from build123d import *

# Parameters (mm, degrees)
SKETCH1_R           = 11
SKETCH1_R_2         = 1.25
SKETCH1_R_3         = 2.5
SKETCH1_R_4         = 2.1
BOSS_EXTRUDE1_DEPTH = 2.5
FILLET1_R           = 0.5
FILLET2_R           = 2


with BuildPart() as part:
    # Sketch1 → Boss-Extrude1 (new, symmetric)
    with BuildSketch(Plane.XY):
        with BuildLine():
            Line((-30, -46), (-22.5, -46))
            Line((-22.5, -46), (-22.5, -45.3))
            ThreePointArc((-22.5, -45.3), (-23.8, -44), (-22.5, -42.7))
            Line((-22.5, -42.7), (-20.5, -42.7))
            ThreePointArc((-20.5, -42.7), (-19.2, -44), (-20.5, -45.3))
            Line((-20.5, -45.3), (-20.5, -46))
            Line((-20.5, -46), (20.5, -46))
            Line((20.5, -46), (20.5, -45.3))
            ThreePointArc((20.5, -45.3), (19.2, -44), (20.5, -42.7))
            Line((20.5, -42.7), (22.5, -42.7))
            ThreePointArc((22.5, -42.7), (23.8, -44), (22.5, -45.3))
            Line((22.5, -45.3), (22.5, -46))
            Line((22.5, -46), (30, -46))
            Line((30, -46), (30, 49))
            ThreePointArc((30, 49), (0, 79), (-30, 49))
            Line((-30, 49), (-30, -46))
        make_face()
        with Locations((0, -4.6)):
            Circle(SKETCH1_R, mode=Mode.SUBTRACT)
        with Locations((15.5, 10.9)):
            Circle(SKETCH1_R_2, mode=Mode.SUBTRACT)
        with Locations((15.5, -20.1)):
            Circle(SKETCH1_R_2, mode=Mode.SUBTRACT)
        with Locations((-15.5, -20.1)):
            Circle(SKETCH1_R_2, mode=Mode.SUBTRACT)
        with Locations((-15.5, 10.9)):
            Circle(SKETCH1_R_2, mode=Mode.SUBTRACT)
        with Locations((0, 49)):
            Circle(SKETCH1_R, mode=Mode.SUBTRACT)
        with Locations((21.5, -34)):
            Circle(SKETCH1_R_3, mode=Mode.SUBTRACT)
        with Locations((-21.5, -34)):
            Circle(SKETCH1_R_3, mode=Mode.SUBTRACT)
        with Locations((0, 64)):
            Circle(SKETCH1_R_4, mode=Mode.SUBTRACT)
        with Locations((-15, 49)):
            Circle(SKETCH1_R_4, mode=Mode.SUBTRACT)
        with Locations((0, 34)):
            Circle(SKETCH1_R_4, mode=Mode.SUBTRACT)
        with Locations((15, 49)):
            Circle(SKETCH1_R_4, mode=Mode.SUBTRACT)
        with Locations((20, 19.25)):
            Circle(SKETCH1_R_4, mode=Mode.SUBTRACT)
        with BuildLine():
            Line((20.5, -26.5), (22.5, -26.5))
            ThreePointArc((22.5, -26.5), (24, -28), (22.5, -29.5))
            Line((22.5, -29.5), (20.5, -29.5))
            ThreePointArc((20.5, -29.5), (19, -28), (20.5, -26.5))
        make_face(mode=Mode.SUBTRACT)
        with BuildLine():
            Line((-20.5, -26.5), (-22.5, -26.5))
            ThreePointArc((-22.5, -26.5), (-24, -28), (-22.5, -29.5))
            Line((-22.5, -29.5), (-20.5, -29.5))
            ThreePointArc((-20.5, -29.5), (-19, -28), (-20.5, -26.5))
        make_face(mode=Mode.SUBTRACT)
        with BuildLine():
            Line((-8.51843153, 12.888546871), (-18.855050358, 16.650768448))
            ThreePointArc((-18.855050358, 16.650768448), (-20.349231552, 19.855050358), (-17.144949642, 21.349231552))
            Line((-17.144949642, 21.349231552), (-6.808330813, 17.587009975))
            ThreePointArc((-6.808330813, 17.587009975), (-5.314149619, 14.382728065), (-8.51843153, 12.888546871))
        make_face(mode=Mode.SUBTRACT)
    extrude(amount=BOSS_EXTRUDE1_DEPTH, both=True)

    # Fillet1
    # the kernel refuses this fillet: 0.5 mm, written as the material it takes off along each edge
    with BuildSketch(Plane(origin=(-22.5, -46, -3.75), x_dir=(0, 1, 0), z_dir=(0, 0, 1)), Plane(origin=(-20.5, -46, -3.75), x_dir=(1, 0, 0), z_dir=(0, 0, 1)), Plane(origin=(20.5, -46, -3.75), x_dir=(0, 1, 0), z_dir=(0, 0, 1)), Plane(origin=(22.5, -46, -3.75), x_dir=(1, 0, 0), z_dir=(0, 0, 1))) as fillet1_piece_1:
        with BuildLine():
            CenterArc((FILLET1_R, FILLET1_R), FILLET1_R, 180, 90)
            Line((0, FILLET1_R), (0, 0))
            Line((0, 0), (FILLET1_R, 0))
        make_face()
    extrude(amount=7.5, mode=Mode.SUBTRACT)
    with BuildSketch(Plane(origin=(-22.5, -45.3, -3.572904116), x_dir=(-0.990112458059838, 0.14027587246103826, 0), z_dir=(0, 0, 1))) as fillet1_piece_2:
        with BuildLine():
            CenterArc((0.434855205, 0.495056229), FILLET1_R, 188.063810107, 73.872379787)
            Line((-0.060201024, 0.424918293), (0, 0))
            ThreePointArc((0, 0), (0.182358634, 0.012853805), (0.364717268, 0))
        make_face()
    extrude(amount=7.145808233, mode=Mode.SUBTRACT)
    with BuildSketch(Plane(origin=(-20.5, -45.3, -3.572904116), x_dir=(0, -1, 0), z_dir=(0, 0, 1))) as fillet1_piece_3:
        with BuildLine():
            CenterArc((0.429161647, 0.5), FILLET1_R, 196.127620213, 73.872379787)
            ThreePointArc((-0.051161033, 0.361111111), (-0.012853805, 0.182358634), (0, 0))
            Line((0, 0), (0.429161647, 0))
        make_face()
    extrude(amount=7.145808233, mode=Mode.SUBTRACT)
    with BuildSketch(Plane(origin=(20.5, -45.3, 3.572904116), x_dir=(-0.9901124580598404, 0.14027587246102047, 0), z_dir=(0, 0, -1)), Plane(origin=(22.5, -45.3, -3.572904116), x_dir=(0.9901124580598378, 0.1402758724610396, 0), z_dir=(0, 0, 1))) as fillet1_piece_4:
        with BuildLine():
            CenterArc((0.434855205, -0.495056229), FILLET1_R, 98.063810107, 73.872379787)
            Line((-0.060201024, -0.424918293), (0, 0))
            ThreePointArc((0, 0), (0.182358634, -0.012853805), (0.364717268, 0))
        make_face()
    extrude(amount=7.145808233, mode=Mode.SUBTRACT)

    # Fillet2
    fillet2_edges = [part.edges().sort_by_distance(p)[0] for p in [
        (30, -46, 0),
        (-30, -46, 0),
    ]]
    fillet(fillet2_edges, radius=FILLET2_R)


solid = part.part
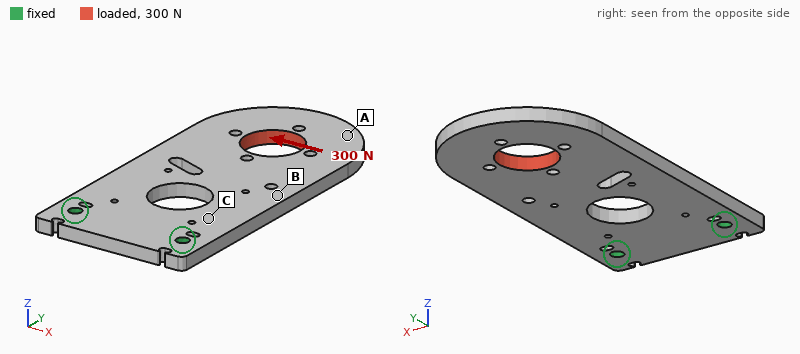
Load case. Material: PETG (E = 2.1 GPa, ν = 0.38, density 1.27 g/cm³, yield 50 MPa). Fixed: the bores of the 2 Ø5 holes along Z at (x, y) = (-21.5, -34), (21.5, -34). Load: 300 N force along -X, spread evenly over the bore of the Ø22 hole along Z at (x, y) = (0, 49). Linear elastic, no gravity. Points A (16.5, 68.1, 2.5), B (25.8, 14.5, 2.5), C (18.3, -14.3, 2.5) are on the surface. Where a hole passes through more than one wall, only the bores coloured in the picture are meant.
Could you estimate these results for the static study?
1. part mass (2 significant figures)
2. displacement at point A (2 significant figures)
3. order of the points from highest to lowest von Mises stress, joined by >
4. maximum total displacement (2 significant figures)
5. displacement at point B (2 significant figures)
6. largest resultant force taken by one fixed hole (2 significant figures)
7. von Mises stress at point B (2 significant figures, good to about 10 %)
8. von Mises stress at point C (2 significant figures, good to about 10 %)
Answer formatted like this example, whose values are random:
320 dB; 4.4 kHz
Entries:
39 g; 0.83 mm; C > B > A; 0.90 mm; 0.38 mm; 570 N; 2.8 MPa; 4.9 MPa
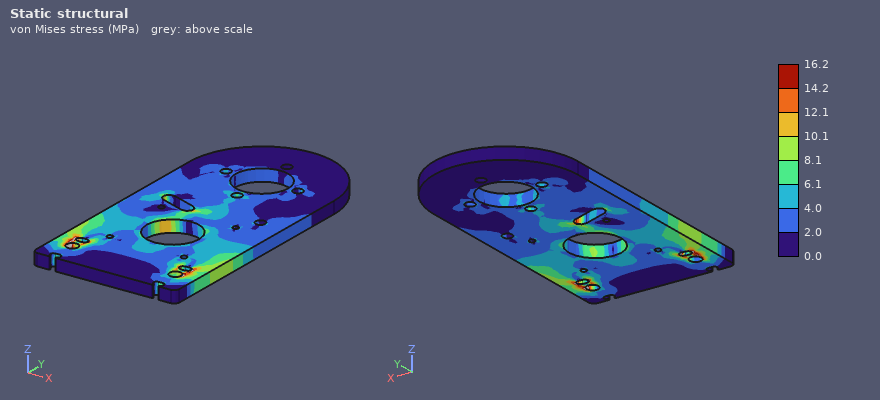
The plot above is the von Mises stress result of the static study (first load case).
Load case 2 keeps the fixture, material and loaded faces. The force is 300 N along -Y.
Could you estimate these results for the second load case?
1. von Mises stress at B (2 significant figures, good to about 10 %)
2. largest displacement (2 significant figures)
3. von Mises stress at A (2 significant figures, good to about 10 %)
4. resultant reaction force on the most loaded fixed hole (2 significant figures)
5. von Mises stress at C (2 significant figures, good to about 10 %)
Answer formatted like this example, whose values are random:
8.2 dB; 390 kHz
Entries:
1.5 MPa; 87 µm; 0.66 MPa; 150 N; 1.5 MPa
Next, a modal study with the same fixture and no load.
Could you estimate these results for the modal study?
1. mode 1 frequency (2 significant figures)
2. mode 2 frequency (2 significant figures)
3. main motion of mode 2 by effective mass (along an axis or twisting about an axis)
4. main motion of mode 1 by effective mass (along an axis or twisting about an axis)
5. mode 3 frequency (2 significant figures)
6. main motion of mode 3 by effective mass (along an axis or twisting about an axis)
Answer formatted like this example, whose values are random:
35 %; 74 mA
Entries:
82 Hz; 330 Hz; twisting about Y; along Z; 490 Hz; along Z
